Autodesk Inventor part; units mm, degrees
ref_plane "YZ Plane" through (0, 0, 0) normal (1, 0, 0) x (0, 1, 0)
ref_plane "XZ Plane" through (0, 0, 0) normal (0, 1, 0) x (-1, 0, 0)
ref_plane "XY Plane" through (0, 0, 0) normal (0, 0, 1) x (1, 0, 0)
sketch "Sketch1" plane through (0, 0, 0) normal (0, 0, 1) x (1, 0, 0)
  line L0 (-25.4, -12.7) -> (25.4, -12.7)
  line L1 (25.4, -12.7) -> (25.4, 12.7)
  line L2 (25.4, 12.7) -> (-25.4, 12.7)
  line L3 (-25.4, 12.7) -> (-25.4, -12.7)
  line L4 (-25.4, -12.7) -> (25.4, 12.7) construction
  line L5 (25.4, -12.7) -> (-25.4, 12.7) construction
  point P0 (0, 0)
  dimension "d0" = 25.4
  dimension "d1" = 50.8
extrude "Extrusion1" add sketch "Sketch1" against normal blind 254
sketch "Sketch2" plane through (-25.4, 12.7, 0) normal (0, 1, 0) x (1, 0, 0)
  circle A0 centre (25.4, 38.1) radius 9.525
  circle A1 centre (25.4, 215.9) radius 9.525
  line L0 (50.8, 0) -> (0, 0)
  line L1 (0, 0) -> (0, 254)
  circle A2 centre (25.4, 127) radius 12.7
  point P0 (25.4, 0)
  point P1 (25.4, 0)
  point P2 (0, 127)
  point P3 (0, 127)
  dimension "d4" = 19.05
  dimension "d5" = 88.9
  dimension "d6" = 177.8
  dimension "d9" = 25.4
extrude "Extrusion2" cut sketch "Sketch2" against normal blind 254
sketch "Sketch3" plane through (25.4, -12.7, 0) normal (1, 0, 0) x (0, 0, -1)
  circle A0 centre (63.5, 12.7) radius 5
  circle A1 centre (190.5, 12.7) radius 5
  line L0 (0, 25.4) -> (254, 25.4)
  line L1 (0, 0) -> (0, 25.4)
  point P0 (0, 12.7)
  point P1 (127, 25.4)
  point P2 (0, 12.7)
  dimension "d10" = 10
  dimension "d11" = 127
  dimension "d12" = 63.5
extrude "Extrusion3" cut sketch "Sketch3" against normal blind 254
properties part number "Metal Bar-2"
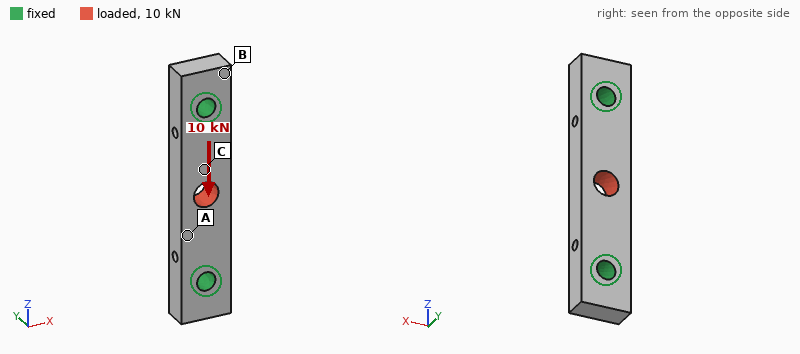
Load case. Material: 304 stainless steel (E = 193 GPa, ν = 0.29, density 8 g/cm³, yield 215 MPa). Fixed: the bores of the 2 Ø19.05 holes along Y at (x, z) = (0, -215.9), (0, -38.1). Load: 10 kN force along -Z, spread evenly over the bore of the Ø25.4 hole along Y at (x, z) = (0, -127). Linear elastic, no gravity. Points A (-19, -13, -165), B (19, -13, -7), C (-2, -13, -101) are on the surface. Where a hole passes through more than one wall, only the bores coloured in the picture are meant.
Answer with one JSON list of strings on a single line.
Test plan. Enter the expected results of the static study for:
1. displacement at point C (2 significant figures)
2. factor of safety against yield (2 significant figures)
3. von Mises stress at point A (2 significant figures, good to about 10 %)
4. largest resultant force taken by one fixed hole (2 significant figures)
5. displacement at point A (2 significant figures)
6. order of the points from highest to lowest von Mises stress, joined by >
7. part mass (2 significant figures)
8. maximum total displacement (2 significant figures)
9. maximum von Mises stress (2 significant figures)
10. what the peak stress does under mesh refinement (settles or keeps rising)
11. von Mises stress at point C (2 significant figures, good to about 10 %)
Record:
["1.5 µm", "15", "3.9 MPa", "5.0 kN", "1.3 µm", "C > A > B", "2.3 kg", "2.1 µm", "15 MPa", "settles", "4.9 MPa"]
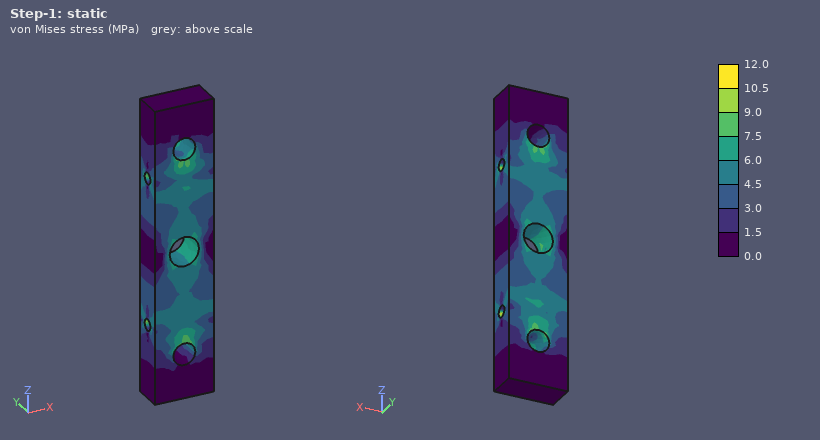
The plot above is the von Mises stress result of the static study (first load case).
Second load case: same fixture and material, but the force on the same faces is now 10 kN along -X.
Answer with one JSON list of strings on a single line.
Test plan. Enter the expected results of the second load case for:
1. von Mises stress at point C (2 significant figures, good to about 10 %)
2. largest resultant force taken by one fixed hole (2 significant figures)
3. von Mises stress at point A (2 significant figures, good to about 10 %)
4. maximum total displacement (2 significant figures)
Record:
["9.8 MPa", "5.0 kN", "6.7 MPa", "13 µm"]
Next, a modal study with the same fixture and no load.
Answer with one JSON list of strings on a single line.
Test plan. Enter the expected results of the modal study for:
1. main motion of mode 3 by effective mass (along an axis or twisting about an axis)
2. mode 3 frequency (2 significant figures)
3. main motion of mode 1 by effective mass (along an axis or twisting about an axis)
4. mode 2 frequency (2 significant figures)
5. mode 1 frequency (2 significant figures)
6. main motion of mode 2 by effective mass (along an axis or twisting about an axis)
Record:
["twisting about Z", "6600 Hz", "along Y", "5300 Hz", "3700 Hz", "along X"]
